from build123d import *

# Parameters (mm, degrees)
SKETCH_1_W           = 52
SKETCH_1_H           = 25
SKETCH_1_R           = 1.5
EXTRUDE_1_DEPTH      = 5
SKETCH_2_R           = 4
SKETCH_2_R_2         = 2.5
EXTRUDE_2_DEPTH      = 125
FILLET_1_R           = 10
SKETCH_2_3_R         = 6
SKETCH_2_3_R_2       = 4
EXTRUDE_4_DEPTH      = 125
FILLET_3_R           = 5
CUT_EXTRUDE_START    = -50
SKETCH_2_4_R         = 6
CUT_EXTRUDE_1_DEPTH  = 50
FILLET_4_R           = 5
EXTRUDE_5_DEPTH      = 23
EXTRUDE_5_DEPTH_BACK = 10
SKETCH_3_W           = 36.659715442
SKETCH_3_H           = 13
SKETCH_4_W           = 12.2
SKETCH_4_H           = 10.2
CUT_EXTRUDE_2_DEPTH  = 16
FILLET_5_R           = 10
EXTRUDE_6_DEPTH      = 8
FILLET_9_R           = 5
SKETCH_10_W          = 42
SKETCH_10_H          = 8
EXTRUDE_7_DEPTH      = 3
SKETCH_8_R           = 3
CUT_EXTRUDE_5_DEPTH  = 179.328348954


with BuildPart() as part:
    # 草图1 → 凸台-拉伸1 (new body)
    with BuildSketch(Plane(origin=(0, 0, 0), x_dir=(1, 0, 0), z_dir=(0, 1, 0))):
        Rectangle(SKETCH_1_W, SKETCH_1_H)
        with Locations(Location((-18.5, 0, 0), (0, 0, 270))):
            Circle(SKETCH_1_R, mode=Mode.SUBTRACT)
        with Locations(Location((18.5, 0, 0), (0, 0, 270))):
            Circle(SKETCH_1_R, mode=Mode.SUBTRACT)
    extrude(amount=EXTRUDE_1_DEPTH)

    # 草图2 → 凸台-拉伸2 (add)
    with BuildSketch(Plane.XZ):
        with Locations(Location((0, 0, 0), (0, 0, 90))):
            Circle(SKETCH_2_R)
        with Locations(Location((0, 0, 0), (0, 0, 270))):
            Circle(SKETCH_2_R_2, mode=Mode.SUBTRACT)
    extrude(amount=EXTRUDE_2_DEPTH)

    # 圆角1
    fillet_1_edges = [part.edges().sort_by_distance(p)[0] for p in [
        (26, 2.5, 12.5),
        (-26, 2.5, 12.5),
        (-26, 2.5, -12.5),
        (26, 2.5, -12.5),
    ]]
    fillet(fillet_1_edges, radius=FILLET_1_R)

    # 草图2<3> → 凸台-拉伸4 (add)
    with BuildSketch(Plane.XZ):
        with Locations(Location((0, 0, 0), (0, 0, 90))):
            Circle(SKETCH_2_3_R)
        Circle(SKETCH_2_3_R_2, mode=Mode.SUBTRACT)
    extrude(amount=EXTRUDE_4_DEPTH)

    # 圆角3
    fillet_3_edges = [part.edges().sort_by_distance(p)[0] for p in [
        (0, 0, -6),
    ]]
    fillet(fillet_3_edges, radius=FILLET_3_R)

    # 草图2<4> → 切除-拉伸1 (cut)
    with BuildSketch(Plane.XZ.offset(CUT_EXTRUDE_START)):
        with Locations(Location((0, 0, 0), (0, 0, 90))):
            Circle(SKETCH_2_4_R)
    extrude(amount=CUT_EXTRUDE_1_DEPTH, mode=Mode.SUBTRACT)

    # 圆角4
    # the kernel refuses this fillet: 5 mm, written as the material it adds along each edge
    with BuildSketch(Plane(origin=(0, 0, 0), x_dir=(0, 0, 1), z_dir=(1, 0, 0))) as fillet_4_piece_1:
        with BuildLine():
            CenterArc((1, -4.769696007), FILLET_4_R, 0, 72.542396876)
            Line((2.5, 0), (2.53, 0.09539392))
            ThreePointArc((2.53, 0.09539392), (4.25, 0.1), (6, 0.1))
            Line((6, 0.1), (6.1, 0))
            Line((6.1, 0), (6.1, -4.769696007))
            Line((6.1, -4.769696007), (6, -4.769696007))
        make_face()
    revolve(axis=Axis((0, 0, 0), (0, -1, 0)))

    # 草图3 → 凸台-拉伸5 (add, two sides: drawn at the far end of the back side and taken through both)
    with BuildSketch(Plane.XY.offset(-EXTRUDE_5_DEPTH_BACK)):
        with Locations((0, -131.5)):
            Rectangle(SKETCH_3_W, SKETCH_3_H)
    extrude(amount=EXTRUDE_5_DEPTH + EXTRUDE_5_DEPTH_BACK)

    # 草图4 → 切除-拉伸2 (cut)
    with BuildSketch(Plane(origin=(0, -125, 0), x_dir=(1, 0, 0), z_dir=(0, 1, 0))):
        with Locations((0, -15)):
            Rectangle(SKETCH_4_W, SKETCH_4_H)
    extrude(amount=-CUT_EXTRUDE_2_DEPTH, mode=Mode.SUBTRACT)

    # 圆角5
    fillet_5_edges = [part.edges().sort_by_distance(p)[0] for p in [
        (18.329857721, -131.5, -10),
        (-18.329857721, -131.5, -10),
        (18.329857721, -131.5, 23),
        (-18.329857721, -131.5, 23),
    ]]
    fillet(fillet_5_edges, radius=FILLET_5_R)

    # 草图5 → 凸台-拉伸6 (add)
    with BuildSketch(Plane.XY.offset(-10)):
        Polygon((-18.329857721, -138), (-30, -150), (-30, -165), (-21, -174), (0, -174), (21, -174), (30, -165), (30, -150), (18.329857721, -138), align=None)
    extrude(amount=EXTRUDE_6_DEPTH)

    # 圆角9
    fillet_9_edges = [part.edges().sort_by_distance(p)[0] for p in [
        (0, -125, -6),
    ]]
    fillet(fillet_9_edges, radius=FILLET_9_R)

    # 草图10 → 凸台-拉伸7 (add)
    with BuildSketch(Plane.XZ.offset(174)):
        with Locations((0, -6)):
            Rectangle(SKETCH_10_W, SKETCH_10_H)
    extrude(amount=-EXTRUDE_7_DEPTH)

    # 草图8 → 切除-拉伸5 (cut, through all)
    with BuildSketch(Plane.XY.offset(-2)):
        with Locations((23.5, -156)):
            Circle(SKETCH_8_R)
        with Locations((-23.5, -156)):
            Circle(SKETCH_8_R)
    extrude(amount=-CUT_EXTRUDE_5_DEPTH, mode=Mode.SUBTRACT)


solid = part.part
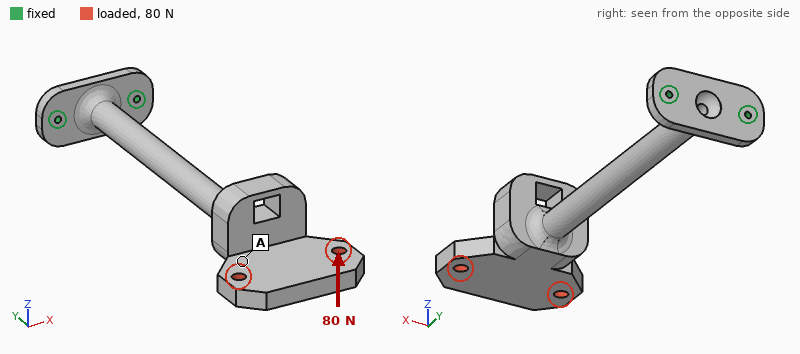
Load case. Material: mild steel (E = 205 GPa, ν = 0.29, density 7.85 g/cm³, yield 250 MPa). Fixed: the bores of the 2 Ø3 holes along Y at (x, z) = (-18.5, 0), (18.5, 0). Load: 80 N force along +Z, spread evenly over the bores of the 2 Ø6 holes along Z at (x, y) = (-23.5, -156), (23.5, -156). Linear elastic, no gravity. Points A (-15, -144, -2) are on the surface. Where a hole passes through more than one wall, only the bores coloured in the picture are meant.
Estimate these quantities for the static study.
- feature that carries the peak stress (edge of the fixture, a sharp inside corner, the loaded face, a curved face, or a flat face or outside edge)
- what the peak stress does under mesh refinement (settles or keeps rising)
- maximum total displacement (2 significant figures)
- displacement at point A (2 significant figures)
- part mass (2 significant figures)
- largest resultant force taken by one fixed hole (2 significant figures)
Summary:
edge of the fixture
keeps rising
0.82 mm
0.64 mm
360 g
40 N
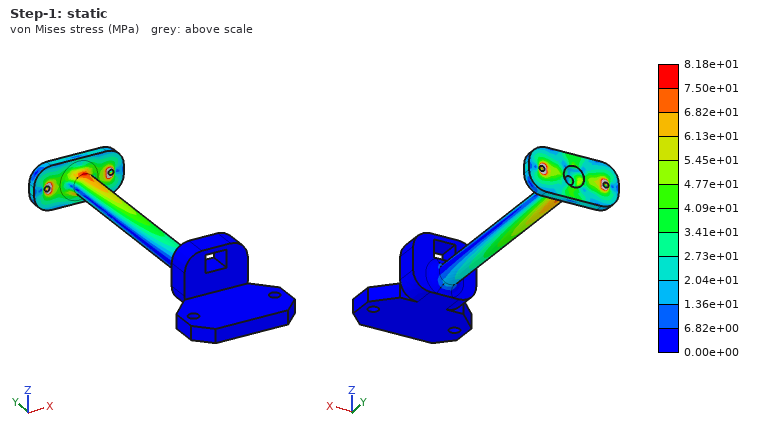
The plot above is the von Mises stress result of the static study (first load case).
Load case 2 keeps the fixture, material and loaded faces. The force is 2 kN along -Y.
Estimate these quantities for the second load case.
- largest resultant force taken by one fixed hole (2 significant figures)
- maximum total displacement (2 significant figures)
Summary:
1.2 kN
1.1 mm
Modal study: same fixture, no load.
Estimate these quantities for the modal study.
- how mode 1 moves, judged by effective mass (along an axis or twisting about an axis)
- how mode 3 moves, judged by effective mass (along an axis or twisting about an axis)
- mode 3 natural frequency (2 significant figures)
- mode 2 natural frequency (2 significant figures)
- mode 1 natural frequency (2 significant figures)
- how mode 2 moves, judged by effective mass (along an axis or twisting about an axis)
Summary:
along Z
twisting about Y
740 Hz
140 Hz
120 Hz
along X
